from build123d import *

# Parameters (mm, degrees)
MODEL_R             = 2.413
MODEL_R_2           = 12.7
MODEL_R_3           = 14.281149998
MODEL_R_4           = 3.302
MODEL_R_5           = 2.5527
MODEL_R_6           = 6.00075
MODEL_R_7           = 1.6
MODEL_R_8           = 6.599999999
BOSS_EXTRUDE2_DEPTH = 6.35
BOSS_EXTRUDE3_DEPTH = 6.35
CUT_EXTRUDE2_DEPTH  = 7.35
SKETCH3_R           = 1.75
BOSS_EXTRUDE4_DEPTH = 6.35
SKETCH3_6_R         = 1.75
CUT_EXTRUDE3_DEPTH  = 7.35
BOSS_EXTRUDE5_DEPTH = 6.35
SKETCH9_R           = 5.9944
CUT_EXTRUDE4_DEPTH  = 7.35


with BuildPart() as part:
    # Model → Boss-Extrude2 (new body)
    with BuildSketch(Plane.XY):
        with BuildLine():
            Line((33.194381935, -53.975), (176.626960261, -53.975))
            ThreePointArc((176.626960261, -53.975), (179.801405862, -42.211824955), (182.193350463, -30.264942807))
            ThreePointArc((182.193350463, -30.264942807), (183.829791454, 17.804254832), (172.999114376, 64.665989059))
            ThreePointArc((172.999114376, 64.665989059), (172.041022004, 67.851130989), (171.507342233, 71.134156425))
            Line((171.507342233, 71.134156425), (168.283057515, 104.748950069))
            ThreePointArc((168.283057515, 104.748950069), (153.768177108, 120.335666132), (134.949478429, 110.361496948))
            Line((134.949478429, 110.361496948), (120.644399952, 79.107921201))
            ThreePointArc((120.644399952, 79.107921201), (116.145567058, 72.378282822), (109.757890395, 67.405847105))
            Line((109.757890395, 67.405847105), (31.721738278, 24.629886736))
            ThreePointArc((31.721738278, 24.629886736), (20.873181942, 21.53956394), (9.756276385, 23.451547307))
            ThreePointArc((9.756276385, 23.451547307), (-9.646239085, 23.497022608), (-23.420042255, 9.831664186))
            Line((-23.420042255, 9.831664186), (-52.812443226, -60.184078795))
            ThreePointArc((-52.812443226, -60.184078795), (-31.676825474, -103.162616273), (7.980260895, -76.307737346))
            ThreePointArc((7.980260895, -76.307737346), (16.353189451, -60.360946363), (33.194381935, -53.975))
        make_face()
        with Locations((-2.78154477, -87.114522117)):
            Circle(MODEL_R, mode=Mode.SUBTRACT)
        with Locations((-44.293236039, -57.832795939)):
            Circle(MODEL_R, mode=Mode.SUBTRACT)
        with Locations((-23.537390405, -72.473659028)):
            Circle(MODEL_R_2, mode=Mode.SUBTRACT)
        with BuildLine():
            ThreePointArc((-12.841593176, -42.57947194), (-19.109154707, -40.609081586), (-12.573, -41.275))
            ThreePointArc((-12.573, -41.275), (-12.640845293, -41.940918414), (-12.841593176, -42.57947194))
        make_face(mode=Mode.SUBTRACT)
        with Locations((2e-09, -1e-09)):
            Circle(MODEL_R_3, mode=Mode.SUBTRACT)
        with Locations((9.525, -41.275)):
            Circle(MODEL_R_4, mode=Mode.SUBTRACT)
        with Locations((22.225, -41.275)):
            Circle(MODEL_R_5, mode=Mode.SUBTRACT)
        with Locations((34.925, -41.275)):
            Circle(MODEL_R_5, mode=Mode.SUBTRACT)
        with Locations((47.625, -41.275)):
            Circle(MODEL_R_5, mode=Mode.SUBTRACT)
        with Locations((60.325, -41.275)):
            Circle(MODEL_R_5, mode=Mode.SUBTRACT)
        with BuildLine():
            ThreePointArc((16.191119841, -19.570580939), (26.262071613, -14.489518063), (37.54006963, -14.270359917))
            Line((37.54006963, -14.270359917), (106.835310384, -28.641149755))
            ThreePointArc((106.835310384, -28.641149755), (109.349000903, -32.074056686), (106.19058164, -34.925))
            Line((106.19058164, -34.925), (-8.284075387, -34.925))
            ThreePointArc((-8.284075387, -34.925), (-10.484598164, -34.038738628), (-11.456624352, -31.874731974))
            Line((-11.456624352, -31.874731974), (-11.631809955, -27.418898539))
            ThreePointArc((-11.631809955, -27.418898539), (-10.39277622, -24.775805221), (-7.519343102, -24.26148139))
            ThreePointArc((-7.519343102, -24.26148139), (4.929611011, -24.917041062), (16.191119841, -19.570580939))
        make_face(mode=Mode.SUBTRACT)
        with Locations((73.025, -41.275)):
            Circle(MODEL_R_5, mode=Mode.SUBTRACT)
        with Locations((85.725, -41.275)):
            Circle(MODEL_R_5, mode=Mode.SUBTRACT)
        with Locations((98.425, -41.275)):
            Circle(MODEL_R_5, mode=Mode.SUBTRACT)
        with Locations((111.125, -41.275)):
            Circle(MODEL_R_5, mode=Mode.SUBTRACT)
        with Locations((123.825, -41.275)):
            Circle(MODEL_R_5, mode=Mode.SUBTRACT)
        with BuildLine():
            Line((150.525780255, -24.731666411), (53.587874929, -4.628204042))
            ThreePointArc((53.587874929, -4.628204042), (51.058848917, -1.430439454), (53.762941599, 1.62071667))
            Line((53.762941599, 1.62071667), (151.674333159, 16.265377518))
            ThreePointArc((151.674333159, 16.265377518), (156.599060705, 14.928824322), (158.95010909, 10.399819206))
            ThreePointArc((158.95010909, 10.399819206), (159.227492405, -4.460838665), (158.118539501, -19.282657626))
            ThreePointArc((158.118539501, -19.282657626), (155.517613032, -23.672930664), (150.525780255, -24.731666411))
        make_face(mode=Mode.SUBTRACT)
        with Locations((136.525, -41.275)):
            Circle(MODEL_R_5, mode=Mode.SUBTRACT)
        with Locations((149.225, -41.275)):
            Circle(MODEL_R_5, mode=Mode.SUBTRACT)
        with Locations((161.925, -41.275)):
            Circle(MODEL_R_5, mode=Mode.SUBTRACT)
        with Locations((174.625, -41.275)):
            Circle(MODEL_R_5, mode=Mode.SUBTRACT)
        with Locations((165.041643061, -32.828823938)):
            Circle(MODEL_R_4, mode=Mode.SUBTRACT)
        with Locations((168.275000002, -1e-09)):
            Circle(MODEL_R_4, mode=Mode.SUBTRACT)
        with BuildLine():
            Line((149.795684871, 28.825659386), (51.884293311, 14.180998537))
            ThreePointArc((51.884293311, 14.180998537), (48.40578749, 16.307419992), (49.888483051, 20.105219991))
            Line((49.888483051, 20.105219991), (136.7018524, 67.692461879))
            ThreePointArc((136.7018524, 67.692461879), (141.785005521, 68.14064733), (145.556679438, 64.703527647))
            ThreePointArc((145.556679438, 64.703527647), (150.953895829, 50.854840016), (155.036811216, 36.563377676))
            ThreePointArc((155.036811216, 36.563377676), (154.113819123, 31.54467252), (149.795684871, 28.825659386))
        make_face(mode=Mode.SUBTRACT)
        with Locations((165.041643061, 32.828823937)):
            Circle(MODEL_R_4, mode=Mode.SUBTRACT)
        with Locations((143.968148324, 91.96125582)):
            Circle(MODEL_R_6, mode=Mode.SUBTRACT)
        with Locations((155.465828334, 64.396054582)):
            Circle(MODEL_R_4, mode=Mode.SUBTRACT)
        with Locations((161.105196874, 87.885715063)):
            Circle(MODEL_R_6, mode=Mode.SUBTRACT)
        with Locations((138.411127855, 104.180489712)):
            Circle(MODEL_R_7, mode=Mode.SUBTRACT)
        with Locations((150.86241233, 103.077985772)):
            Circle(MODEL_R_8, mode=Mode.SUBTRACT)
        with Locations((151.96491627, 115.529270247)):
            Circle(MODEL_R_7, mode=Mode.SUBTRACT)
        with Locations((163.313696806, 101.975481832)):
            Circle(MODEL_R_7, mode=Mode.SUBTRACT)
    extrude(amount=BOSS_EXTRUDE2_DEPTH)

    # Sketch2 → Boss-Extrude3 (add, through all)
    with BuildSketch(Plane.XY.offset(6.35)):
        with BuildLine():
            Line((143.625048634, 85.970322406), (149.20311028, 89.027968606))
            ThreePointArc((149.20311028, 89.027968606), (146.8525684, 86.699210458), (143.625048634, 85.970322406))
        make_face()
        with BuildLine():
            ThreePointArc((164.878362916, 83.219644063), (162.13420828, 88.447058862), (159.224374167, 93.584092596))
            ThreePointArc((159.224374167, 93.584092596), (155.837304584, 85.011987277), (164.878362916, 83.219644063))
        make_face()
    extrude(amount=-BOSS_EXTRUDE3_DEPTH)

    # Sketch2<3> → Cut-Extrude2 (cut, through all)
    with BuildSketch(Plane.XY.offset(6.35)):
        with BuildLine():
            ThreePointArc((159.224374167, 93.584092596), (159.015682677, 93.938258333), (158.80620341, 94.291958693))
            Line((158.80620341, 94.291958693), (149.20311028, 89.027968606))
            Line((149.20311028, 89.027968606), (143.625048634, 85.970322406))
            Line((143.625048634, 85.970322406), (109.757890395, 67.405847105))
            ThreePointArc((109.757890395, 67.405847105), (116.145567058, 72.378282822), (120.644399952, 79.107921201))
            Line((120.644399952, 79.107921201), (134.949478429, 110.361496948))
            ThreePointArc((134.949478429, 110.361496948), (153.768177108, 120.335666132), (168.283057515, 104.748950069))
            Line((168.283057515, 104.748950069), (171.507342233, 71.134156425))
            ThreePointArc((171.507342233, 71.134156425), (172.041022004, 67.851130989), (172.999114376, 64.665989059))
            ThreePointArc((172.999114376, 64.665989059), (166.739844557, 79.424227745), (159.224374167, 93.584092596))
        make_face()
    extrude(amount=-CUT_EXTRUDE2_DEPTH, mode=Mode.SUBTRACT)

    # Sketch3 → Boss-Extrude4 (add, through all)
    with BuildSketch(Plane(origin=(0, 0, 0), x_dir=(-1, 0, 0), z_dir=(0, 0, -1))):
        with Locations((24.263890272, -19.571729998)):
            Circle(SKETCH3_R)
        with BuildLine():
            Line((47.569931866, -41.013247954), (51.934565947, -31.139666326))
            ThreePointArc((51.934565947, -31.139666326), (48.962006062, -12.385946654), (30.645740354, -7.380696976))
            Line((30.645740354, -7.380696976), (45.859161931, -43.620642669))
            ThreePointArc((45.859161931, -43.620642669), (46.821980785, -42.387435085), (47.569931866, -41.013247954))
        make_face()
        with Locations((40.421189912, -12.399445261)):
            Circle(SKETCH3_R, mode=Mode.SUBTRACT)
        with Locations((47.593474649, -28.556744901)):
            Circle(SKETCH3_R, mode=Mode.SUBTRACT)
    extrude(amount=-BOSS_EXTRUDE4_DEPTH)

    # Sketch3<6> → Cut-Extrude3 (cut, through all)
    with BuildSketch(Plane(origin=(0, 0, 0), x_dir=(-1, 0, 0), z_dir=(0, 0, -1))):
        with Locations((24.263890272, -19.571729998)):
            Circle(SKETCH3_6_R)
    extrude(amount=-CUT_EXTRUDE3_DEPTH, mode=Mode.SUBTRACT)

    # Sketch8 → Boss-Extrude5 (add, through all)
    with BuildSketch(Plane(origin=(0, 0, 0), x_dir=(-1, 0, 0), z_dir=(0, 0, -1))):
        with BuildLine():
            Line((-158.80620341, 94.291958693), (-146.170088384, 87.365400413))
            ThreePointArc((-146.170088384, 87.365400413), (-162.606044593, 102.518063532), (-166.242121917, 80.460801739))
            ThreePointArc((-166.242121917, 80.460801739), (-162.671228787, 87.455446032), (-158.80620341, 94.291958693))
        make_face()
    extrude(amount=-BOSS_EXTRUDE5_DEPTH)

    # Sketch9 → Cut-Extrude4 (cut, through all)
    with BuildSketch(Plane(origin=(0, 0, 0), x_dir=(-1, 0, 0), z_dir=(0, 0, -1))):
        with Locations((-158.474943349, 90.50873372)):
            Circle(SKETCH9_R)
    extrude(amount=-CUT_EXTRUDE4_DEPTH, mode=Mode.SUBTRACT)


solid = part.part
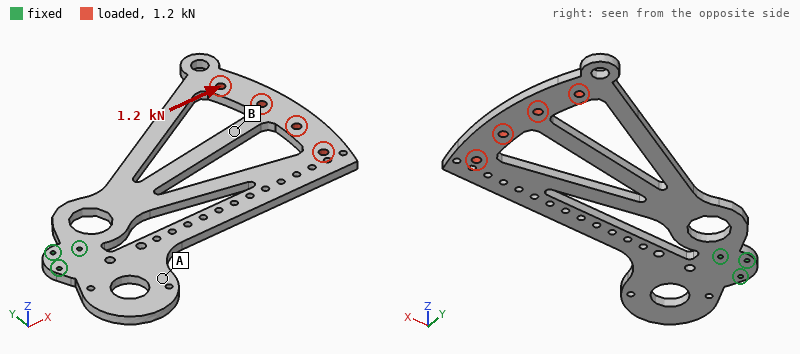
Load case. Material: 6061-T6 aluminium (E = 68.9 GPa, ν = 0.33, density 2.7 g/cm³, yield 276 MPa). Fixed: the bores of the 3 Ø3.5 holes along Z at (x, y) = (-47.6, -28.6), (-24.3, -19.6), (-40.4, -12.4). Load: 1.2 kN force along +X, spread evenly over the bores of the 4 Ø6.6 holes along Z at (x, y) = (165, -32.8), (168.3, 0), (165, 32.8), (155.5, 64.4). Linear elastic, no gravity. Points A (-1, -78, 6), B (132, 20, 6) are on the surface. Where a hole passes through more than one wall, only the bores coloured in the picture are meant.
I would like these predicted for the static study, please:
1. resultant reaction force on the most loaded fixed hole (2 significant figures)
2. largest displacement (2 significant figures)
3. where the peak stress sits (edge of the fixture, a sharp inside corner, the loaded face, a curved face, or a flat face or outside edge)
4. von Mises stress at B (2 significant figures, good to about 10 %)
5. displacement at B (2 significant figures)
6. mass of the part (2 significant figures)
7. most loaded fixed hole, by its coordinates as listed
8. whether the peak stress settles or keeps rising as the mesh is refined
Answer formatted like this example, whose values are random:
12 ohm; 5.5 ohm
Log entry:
1.5 kN; 0.30 mm; edge of the fixture; 8.6 MPa; 0.22 mm; 300 g; (-24.3, -19.6); keeps rising
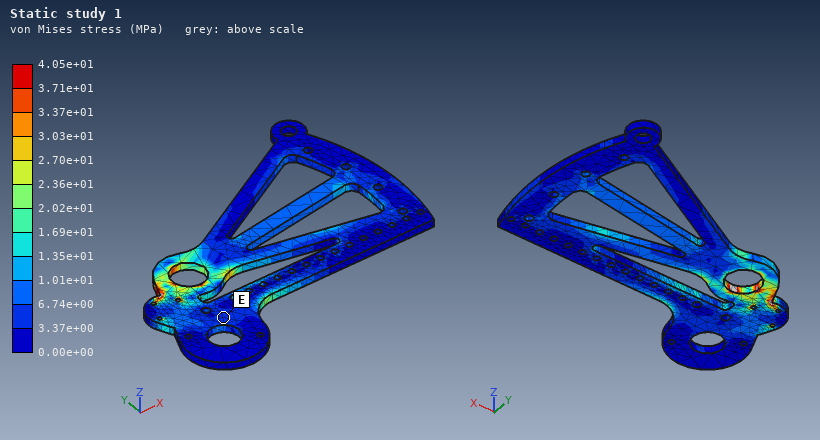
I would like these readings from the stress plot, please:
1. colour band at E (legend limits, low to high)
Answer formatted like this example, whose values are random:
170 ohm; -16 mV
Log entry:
3.37e+00 to 6.74e+00 MPa
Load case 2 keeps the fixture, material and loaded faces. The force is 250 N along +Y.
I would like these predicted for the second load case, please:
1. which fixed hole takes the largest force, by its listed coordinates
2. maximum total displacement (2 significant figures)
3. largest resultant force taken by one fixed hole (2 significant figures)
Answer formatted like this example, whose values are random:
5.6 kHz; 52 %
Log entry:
(-24.3, -19.6); 0.27 mm; 1.7 kN
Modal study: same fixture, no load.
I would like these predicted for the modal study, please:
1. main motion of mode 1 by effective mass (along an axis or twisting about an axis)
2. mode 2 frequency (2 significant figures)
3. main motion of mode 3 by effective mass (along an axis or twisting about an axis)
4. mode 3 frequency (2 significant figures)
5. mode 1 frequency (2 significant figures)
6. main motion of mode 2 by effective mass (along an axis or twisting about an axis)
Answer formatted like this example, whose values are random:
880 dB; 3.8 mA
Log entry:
along Z; 240 Hz; along Y; 470 Hz; 82 Hz; twisting about X
